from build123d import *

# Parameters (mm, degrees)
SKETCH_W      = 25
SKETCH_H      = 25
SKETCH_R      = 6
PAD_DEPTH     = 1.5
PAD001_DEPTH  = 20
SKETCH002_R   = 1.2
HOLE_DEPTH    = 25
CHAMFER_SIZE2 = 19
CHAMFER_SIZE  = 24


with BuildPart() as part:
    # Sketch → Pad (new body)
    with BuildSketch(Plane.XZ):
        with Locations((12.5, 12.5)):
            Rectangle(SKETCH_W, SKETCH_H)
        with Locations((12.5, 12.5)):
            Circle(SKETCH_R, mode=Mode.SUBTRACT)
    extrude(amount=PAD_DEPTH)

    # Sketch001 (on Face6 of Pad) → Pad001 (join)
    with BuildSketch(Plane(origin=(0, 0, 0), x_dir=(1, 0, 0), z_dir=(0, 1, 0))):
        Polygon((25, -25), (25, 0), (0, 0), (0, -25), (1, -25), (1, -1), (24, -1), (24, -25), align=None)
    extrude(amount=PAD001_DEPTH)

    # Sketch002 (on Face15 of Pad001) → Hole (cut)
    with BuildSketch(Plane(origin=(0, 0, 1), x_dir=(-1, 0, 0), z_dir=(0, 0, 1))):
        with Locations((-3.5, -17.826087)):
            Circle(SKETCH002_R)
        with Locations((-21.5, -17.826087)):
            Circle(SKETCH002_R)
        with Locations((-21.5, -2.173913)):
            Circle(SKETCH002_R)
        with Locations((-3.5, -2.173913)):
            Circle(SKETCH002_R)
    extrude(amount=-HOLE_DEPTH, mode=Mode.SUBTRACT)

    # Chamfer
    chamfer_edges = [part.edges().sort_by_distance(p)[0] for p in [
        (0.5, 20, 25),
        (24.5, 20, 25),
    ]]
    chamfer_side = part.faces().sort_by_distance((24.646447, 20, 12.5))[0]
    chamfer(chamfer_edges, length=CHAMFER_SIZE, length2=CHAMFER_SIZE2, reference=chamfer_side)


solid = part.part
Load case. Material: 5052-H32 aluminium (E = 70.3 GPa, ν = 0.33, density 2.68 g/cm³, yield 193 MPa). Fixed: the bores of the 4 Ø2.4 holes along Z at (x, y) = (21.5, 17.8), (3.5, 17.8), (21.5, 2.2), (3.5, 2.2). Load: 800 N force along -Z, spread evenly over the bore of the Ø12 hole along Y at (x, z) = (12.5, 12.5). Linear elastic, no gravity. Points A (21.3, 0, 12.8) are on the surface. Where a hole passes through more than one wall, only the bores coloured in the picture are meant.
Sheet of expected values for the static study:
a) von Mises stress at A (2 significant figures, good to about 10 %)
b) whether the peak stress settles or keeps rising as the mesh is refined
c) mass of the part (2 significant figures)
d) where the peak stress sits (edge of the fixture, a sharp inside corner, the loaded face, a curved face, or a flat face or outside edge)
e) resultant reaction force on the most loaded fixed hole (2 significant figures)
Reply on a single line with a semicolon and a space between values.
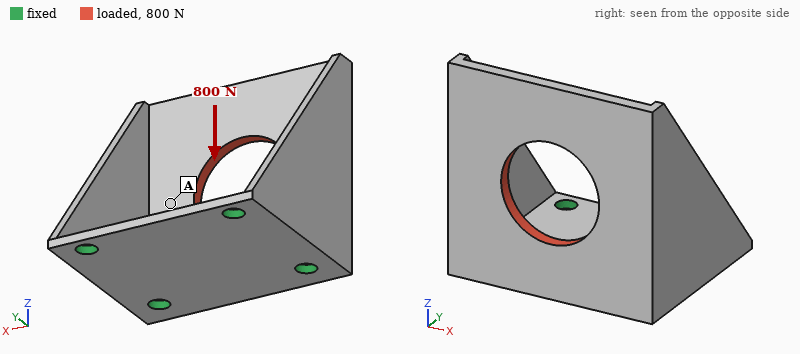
26 MPa; keeps rising; 4.7 g; edge of the fixture; 440 N
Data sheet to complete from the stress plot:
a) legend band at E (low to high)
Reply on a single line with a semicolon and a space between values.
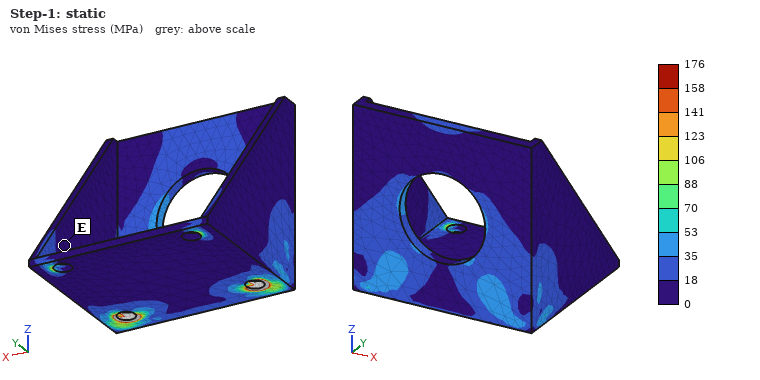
0 to 18 MPa
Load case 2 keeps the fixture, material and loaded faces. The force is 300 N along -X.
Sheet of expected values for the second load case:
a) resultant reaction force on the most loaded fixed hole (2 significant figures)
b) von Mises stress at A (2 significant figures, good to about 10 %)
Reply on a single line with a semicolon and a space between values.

250 N; 23 MPa
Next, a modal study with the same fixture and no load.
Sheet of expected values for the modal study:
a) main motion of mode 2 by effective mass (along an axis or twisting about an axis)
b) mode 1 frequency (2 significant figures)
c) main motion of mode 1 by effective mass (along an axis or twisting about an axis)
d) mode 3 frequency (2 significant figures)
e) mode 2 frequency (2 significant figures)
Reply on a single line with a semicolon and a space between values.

along X; 6100 Hz; along Y; 11 kHz; 8600 Hz
